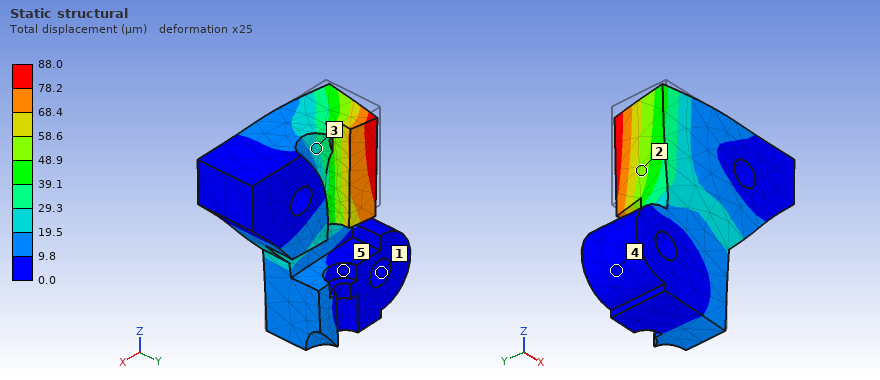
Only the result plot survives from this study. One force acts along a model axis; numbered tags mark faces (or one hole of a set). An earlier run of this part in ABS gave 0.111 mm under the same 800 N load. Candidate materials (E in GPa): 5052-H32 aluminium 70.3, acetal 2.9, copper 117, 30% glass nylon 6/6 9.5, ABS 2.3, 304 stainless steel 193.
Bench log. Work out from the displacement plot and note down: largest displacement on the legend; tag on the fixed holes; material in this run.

88.0 µm
1
acetal
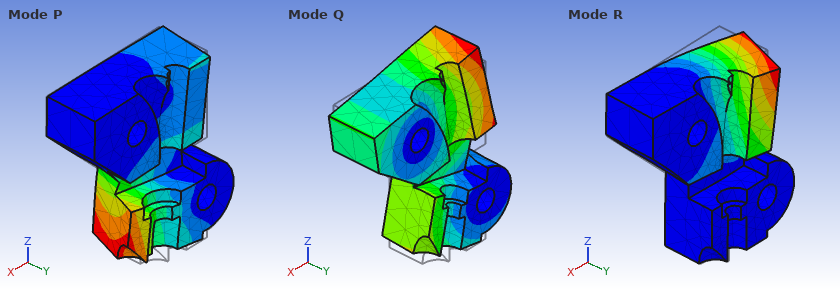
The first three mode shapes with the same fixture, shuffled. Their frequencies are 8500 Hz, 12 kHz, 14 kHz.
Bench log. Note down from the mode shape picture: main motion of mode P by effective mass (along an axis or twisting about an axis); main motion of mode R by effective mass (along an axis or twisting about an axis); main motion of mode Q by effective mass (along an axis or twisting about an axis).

along Y
along Y
along Z
